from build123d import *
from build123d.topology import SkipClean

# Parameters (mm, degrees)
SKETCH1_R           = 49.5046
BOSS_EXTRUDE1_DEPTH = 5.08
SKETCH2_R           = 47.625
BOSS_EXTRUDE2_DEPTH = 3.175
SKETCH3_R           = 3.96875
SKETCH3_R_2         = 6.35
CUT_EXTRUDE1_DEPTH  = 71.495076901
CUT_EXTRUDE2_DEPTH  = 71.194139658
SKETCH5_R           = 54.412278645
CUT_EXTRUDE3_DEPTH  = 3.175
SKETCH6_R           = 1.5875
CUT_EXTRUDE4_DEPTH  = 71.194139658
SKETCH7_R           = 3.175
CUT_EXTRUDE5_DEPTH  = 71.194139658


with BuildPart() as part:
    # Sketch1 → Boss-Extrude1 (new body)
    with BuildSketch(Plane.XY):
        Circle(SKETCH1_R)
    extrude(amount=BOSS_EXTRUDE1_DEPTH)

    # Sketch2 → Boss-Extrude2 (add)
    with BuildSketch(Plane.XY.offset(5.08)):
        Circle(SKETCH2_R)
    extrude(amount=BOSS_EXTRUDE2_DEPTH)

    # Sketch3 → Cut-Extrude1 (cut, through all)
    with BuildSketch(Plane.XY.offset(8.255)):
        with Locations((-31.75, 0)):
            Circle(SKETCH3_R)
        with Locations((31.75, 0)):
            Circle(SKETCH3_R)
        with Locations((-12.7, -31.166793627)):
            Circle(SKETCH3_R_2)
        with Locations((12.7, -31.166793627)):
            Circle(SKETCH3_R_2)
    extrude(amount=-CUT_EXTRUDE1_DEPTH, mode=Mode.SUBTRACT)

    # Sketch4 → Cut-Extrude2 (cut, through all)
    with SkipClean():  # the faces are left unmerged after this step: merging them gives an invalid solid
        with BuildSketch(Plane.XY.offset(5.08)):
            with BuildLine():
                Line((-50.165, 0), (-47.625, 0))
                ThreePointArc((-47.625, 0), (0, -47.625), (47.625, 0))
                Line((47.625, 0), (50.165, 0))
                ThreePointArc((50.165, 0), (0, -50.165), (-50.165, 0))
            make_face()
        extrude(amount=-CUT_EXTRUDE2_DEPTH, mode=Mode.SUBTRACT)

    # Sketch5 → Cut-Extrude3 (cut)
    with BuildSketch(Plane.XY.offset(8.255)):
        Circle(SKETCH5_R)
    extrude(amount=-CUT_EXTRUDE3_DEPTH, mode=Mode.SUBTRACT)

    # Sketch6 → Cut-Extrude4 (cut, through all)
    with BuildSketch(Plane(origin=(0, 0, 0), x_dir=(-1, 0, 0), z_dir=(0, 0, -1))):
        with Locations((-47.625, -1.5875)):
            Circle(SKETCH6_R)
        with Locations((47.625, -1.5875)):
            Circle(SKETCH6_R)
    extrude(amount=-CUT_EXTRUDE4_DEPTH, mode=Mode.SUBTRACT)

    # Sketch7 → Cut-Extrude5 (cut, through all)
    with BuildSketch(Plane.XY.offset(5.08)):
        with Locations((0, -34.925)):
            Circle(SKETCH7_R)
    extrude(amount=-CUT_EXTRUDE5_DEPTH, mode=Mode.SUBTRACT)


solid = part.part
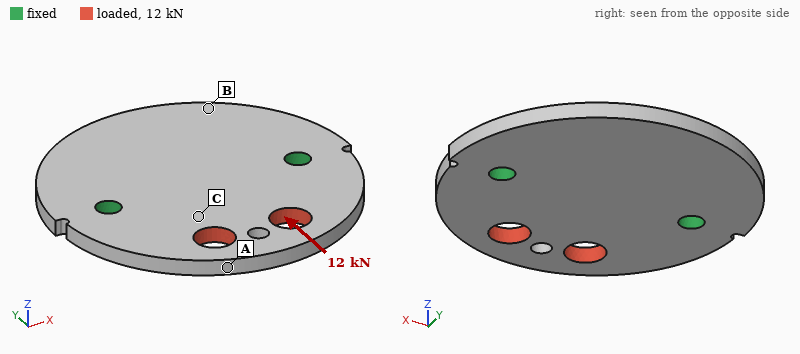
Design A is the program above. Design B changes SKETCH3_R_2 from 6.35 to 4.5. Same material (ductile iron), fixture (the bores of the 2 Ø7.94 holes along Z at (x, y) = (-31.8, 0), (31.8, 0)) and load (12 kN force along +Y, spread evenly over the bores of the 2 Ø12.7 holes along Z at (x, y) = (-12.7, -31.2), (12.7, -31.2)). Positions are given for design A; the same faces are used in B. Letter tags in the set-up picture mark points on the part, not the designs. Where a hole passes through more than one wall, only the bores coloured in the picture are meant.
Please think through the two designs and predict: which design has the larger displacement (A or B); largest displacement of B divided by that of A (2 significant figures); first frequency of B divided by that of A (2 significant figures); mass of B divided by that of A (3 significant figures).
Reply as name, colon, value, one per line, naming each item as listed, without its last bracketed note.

which design has the larger displacement: A
largest displacement of B divided by that of A: 0.92
first frequency of B divided by that of A: 0.99
mass of B divided by that of A: 1.02
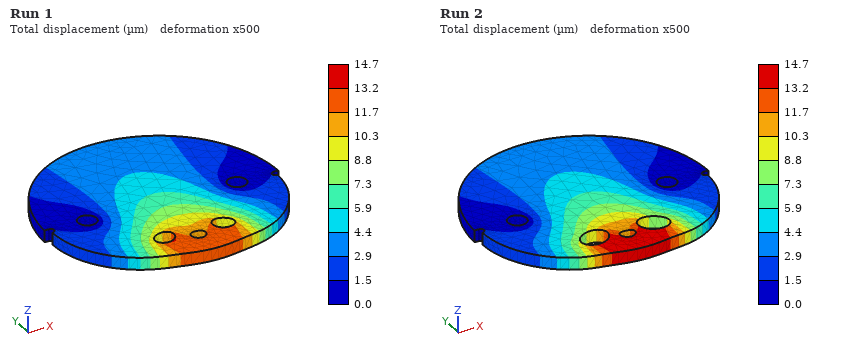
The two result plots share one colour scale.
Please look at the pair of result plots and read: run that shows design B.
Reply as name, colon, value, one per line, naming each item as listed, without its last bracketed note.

run that shows design B: Run 1
